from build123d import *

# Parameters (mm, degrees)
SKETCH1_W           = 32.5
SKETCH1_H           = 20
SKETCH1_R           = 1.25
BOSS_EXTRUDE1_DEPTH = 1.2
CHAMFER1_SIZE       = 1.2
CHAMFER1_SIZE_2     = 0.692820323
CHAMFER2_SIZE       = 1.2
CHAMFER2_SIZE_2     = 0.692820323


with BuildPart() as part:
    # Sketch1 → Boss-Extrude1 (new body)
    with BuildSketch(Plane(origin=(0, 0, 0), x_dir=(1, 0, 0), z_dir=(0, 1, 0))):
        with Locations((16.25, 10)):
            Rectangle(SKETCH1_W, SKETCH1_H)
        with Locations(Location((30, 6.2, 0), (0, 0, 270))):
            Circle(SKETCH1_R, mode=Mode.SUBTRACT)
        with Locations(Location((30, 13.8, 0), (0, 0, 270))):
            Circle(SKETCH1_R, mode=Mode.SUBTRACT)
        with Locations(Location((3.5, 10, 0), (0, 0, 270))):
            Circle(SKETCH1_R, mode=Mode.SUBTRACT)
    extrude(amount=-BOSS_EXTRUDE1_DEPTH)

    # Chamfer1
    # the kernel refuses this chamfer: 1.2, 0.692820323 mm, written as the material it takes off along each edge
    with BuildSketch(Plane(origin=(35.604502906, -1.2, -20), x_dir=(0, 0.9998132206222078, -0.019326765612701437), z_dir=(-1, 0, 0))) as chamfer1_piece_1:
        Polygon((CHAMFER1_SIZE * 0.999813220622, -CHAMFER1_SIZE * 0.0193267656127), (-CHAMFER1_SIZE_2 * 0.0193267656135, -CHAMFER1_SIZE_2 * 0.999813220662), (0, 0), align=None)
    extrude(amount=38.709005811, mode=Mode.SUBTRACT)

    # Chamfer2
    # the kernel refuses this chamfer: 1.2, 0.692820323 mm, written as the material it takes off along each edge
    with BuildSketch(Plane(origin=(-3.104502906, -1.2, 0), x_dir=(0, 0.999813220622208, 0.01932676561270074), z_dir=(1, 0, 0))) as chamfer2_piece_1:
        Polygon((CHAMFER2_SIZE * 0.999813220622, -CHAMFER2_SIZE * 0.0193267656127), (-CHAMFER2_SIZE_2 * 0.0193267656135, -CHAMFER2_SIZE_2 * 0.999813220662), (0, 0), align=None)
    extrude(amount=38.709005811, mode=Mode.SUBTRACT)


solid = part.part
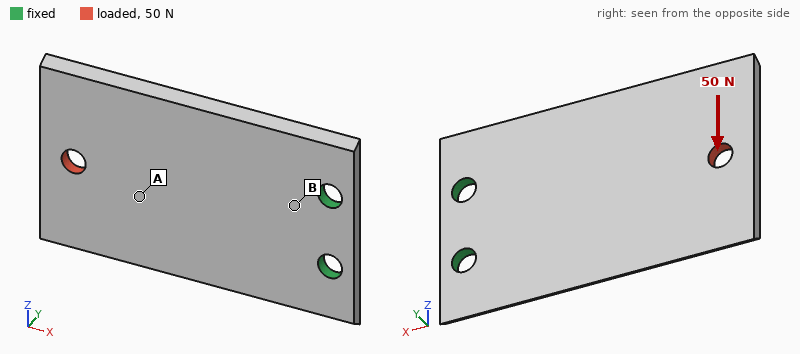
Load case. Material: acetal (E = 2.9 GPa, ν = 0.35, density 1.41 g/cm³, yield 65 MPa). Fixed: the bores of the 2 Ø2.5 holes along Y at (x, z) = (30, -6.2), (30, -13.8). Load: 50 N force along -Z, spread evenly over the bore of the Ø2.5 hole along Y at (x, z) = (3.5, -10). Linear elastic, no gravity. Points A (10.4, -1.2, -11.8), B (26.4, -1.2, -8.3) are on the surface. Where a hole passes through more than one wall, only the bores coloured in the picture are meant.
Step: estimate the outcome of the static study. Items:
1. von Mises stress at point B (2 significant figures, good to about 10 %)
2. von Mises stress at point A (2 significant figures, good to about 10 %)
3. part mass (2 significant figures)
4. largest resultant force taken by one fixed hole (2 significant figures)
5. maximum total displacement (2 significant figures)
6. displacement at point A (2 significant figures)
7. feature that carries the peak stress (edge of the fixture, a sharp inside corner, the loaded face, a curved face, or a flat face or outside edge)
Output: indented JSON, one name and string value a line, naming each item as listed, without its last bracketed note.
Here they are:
{
  "von Mises stress at point B": "14 MPa",
  "von Mises stress at point A": "5.3 MPa",
  "part mass": "1.0 g",
  "largest resultant force taken by one fixed hole": "130 N",
  "maximum total displacement": "0.40 mm",
  "displacement at point A": "0.23 mm",
  "feature that carries the peak stress": "edge of the fixture"
}
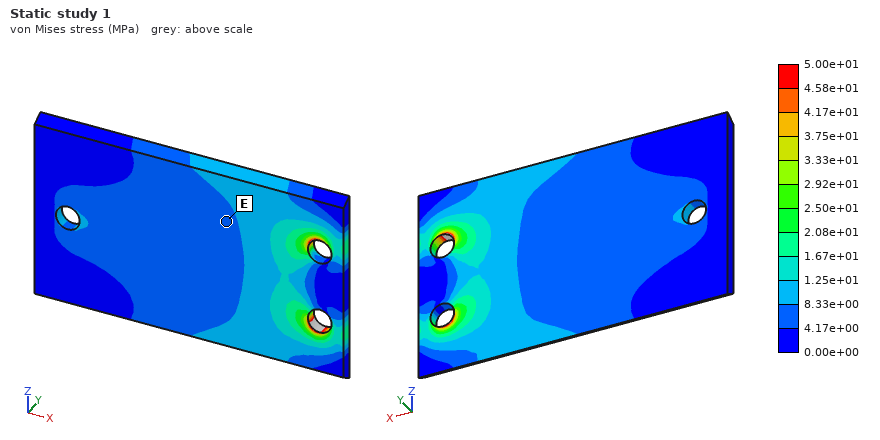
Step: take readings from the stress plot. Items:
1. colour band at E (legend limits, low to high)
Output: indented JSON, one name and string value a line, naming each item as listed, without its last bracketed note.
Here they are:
{
  "colour band at E": "4.17e+00 to 8.33e+00 MPa"
}
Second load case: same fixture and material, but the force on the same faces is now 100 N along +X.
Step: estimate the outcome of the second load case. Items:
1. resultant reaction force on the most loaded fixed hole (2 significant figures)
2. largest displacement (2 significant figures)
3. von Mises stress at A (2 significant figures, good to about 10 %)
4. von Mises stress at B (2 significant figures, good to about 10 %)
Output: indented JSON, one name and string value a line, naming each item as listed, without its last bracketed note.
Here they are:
{
  "resultant reaction force on the most loaded fixed hole": "50 N",
  "largest displacement": "71 µm",
  "von Mises stress at A": "6.9 MPa",
  "von Mises stress at B": "5.0 MPa"
}
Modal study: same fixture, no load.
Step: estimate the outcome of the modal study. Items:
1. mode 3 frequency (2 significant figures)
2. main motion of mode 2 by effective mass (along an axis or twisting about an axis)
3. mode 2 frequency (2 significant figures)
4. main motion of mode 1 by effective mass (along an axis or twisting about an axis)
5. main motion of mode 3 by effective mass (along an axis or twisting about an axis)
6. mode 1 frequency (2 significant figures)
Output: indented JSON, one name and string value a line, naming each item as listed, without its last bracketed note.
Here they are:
{
  "mode 3 frequency": "2000 Hz",
  "main motion of mode 2 by effective mass": "twisting about X",
  "mode 2 frequency": "1000 Hz",
  "main motion of mode 1 by effective mass": "along Y",
  "main motion of mode 3 by effective mass": "along Y",
  "mode 1 frequency": "330 Hz"
}
